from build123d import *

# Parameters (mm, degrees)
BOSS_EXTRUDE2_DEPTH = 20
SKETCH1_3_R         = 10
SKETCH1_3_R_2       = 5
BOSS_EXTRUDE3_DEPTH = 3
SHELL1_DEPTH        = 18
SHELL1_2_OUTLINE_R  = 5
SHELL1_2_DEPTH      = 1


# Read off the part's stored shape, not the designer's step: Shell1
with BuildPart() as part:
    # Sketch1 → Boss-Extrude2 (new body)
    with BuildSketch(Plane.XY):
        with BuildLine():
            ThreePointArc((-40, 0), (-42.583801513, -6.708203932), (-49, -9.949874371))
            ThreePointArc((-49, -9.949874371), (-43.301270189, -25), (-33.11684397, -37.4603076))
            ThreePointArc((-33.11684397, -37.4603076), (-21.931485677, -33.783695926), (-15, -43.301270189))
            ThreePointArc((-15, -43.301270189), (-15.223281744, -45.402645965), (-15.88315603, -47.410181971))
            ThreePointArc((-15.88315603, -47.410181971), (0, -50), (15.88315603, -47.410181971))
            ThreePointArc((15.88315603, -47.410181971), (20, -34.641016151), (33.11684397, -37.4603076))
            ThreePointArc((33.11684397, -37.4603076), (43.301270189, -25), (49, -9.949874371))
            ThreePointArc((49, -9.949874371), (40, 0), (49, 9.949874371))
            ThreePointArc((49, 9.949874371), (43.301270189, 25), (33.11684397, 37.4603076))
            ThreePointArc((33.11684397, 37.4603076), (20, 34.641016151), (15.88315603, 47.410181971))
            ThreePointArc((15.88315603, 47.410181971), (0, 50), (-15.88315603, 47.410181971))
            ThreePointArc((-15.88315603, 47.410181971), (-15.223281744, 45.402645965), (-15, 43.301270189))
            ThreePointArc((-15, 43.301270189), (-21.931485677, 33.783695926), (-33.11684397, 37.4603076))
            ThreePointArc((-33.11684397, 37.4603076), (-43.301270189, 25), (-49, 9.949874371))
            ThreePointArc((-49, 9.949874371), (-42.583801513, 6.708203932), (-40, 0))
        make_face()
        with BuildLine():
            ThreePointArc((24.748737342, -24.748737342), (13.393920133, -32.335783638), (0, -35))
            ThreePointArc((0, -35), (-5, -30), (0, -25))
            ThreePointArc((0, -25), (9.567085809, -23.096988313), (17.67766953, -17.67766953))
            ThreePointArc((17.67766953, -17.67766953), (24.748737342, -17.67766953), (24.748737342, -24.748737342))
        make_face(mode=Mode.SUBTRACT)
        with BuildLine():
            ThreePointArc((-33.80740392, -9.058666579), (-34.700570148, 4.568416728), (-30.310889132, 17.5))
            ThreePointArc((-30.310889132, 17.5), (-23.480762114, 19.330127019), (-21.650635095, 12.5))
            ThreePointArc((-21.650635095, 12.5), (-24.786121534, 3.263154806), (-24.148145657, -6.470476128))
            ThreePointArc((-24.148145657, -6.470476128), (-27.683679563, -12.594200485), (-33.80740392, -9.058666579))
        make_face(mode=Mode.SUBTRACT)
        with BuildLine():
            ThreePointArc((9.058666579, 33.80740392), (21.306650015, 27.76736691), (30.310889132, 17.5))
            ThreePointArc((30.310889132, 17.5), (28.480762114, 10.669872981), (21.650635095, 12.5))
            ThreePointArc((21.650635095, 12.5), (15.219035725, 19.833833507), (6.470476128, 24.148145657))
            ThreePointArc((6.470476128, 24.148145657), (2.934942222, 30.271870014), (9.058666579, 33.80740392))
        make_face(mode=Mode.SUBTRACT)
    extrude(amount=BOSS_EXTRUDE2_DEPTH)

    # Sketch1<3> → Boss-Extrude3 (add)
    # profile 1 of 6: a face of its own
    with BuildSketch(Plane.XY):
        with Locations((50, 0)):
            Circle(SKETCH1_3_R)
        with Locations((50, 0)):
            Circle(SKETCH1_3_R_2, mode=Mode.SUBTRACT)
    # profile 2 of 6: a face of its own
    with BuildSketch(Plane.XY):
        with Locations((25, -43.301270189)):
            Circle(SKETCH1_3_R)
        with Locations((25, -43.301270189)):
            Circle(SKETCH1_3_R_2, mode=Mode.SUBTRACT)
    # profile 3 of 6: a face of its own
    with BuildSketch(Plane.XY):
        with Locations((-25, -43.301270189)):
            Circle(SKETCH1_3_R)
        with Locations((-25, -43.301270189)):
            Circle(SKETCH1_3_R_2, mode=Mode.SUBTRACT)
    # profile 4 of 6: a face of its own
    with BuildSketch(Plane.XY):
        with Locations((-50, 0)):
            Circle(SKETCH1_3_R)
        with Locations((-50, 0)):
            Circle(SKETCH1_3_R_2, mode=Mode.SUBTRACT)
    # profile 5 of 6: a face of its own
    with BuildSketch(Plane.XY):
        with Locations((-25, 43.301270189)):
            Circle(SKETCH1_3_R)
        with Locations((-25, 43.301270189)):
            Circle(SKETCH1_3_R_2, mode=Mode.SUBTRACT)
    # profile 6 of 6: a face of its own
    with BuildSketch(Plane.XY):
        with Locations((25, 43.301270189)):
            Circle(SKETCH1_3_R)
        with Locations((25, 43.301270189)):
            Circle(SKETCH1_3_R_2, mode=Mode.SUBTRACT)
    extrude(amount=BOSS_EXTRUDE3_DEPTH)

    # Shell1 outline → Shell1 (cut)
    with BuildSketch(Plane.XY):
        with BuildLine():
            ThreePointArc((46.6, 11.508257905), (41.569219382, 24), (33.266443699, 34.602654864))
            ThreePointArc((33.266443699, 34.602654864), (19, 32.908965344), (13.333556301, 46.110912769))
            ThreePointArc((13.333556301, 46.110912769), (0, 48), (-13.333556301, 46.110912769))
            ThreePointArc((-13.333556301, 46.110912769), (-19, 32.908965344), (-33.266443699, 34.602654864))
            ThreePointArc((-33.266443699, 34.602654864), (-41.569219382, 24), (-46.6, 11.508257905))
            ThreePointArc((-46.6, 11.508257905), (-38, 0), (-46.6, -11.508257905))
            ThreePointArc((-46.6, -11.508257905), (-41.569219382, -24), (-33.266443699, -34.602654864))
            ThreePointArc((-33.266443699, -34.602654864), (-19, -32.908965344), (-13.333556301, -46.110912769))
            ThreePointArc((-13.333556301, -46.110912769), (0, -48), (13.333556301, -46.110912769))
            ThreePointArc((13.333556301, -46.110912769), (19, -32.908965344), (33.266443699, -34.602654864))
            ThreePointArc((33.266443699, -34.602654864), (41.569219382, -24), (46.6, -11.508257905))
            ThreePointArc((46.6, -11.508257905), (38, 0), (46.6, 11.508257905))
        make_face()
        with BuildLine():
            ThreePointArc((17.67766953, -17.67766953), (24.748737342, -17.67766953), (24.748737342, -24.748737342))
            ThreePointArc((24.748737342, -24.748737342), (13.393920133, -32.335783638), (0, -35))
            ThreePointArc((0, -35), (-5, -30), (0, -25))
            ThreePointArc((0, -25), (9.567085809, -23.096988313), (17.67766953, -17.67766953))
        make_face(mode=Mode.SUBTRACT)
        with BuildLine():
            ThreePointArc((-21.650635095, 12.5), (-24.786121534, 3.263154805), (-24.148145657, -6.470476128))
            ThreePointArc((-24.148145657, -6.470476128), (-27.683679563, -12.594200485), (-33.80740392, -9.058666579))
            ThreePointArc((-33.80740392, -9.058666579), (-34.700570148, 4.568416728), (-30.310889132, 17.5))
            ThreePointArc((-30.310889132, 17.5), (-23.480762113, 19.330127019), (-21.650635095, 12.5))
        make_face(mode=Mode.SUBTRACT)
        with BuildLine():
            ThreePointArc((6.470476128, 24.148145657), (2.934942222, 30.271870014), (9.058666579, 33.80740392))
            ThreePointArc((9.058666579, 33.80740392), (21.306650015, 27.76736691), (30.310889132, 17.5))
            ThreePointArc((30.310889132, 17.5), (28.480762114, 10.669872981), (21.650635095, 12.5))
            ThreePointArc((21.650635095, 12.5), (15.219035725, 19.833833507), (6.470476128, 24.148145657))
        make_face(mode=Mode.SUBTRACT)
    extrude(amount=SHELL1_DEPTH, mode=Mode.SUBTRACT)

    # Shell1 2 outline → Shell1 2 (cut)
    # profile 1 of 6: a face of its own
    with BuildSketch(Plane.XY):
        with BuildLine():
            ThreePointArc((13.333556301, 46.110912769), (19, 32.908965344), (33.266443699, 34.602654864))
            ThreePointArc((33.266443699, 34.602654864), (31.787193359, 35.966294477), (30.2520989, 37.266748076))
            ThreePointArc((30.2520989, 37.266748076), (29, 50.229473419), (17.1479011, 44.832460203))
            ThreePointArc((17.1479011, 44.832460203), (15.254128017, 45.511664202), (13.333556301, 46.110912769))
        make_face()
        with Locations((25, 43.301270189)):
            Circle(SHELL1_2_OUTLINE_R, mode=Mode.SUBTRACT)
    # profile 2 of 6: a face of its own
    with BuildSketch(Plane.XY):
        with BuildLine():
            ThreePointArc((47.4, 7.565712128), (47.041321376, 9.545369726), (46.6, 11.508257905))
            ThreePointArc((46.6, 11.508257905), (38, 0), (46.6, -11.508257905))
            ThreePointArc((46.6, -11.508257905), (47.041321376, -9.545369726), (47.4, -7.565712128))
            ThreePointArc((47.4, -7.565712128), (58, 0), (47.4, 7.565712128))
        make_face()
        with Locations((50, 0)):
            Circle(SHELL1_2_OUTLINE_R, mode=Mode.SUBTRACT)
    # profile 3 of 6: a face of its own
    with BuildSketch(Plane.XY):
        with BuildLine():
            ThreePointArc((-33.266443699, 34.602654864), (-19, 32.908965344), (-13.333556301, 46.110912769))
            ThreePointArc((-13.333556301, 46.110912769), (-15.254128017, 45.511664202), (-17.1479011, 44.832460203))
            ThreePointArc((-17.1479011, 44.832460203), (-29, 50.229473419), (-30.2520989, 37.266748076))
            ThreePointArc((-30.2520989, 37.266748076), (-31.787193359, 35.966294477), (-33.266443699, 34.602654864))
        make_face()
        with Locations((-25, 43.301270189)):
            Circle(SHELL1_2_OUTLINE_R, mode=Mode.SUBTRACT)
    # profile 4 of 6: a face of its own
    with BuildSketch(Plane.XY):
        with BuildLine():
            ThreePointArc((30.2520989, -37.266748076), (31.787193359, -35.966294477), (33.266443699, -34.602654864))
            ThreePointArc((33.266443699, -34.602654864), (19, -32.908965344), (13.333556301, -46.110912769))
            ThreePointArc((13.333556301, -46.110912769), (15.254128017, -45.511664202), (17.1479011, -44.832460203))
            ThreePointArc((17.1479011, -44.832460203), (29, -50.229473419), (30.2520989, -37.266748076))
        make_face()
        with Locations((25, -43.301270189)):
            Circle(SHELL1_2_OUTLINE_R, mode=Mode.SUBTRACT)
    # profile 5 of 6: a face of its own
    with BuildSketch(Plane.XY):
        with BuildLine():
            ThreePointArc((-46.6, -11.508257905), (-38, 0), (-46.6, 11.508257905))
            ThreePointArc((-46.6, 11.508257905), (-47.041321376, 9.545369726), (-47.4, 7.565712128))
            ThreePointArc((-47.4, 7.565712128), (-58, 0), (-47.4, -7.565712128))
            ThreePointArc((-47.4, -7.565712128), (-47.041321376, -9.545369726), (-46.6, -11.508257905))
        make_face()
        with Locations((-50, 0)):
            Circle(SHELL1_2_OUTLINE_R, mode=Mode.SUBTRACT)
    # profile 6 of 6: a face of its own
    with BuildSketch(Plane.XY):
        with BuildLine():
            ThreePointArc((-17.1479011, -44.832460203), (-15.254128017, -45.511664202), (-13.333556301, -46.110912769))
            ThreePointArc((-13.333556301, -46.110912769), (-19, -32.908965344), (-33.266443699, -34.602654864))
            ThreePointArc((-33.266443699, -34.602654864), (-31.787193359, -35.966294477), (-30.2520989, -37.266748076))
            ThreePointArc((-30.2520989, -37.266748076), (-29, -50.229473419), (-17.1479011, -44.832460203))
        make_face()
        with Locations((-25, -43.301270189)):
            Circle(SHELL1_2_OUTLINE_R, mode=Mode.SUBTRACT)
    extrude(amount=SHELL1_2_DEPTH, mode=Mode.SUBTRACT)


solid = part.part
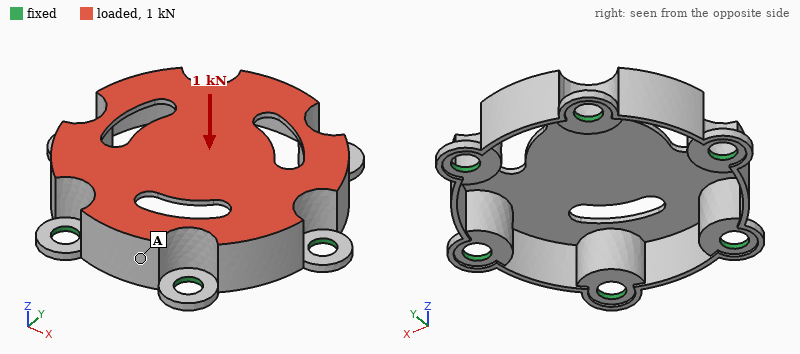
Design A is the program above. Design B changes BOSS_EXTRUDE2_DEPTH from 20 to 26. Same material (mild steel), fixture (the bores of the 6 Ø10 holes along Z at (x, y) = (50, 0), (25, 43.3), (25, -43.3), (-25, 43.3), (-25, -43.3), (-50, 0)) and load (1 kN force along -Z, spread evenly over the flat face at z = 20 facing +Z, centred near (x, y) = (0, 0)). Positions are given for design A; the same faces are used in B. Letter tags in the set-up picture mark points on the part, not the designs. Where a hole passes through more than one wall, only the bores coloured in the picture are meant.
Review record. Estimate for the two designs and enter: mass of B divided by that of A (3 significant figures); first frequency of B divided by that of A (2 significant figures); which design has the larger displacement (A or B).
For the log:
2.30
2.2
A
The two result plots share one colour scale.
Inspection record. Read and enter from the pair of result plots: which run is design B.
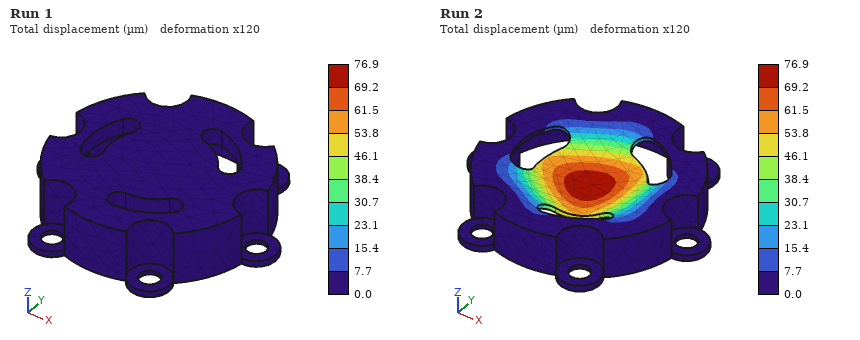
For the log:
Run 1
